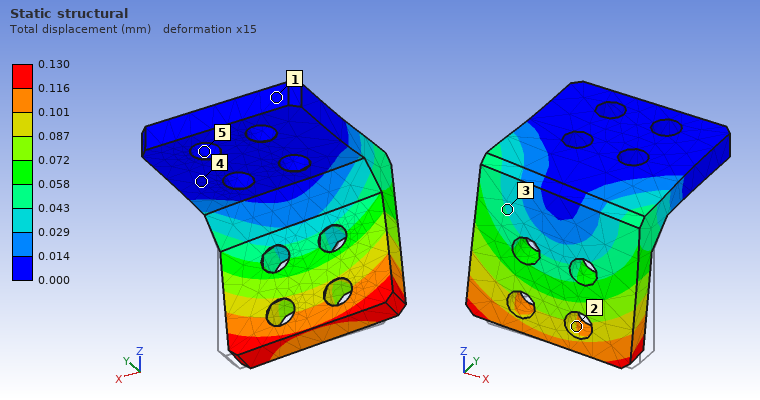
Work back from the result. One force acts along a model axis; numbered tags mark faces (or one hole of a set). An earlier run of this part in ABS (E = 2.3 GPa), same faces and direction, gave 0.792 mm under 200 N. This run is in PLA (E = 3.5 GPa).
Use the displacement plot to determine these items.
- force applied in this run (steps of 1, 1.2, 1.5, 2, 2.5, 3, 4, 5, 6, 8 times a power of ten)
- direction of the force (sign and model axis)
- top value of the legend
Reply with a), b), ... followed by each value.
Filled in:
a) 50 N
b) -X
c) 0.130 mm
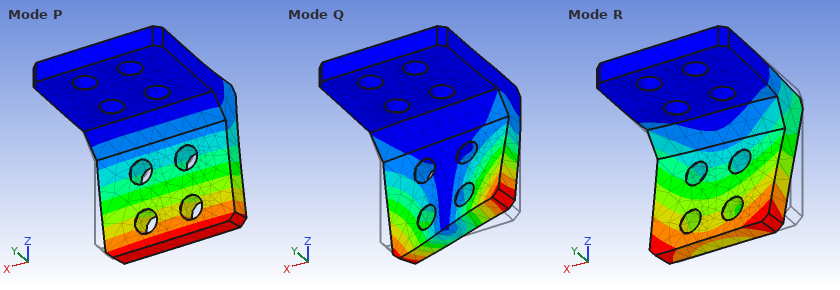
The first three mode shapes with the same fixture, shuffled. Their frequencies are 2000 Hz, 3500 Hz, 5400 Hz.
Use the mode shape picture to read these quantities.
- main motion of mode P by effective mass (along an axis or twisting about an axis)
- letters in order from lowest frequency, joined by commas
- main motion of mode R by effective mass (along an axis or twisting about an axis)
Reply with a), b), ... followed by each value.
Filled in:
a) along Y
b) P, R, Q
c) along X
